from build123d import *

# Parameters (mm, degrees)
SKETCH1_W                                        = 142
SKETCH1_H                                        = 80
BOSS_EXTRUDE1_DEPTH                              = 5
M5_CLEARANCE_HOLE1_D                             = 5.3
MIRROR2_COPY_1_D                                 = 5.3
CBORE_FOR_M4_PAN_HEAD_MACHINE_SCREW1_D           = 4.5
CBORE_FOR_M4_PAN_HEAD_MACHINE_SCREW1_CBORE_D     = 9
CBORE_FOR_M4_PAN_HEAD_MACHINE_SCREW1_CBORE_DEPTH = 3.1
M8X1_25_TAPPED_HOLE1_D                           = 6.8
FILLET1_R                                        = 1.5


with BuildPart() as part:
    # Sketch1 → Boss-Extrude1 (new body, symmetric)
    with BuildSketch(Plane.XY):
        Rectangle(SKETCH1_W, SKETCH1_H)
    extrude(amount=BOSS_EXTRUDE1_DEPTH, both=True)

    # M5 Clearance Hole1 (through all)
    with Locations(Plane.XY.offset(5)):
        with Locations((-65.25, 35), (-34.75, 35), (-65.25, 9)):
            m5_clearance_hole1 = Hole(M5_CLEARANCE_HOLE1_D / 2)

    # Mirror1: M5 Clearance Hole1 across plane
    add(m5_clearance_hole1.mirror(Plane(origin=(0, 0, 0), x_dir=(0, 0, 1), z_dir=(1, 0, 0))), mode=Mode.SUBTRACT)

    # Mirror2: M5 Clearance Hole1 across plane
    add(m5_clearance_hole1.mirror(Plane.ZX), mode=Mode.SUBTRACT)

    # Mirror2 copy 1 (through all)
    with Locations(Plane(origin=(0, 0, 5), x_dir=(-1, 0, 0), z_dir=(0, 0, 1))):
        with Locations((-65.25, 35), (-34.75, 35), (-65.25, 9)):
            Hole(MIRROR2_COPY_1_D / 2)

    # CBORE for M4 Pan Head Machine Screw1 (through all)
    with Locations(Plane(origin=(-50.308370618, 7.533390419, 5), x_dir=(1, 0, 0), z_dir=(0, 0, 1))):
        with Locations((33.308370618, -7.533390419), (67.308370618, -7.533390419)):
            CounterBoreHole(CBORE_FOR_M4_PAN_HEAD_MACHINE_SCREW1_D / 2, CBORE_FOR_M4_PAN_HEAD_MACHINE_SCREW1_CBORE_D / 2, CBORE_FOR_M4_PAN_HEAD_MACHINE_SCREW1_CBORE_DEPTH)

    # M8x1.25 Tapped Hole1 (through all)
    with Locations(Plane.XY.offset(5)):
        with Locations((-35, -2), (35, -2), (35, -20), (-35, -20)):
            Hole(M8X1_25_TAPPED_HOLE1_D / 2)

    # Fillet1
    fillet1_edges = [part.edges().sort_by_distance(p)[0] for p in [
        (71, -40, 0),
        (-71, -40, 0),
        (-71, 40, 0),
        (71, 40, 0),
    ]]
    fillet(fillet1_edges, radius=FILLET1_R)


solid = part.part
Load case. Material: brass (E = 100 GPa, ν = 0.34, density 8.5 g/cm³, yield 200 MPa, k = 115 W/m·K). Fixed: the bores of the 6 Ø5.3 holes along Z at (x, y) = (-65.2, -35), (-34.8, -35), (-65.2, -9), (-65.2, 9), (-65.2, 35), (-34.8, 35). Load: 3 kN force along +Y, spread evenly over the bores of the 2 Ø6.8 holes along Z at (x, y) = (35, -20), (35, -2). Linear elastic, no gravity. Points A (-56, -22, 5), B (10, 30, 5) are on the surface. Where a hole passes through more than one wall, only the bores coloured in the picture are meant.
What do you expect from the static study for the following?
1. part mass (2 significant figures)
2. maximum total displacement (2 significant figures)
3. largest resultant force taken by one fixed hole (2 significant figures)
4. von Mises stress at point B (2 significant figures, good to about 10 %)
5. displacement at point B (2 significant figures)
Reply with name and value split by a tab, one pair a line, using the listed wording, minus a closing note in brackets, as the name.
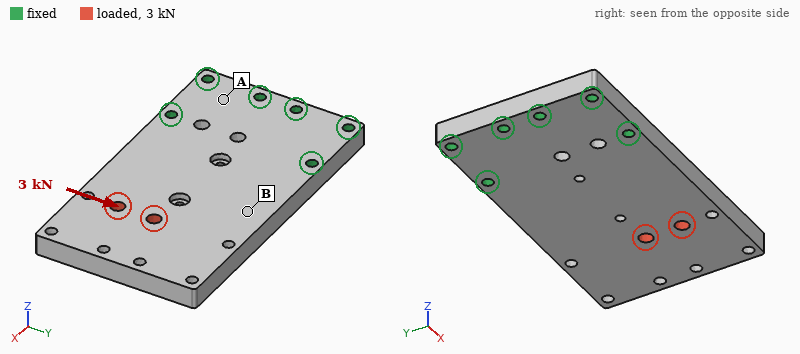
part mass	930 g
maximum total displacement	25 µm
largest resultant force taken by one fixed hole	3.0 kN
von Mises stress at point B	7.0 MPa
displacement at point B	11 µm
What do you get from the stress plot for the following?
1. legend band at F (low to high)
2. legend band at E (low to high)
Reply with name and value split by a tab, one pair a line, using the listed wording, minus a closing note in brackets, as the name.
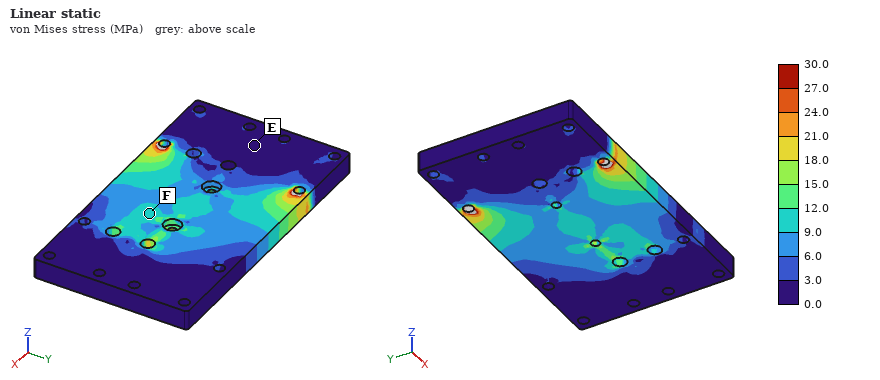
legend band at F	9.0 to 12.0 MPa
legend band at E	0.0 to 3.0 MPa
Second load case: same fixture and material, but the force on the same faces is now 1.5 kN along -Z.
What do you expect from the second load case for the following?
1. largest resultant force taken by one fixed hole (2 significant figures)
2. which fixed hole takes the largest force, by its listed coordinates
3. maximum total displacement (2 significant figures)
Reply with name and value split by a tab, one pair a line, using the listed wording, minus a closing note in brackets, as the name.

largest resultant force taken by one fixed hole	1.7 kN
which fixed hole takes the largest force, by its listed coordinates	(-34.8, -35)
maximum total displacement	0.60 mm
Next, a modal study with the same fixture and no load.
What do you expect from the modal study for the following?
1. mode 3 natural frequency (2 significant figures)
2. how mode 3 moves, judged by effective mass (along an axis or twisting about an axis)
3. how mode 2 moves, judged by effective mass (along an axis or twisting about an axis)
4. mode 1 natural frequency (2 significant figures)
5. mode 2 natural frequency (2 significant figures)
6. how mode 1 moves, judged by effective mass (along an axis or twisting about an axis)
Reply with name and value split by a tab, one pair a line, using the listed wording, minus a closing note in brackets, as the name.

mode 3 natural frequency	2700 Hz
how mode 3 moves, judged by effective mass	along Z
how mode 2 moves, judged by effective mass	twisting about X
mode 1 natural frequency	460 Hz
mode 2 natural frequency	1400 Hz
how mode 1 moves, judged by effective mass	along Z
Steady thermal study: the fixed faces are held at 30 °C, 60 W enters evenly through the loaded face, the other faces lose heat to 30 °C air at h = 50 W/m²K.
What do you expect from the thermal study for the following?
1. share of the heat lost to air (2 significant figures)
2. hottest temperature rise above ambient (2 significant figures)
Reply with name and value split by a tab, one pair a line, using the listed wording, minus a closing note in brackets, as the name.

share of the heat lost to air	41 %
hottest temperature rise above ambient	43 K
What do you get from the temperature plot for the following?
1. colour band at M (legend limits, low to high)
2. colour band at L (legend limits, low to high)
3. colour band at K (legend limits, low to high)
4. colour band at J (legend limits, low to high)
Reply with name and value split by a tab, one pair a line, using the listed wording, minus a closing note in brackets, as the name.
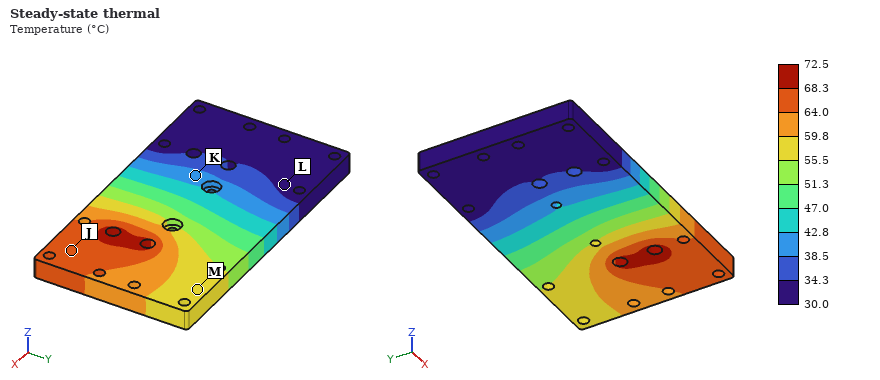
colour band at M	55.5 to 59.8 °C
colour band at L	30.0 to 34.3 °C
colour band at K	38.5 to 42.8 °C
colour band at J	64.0 to 68.3 °C
